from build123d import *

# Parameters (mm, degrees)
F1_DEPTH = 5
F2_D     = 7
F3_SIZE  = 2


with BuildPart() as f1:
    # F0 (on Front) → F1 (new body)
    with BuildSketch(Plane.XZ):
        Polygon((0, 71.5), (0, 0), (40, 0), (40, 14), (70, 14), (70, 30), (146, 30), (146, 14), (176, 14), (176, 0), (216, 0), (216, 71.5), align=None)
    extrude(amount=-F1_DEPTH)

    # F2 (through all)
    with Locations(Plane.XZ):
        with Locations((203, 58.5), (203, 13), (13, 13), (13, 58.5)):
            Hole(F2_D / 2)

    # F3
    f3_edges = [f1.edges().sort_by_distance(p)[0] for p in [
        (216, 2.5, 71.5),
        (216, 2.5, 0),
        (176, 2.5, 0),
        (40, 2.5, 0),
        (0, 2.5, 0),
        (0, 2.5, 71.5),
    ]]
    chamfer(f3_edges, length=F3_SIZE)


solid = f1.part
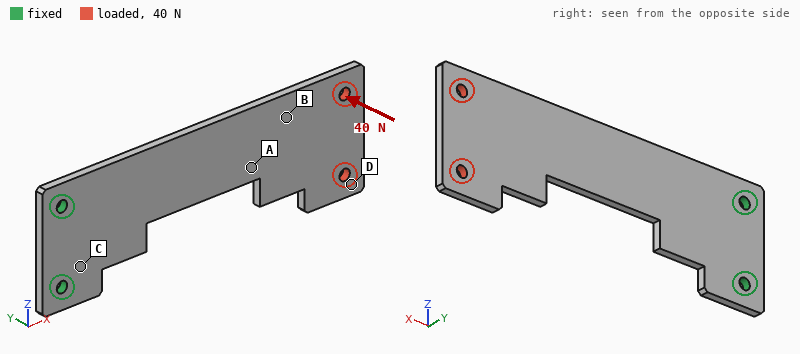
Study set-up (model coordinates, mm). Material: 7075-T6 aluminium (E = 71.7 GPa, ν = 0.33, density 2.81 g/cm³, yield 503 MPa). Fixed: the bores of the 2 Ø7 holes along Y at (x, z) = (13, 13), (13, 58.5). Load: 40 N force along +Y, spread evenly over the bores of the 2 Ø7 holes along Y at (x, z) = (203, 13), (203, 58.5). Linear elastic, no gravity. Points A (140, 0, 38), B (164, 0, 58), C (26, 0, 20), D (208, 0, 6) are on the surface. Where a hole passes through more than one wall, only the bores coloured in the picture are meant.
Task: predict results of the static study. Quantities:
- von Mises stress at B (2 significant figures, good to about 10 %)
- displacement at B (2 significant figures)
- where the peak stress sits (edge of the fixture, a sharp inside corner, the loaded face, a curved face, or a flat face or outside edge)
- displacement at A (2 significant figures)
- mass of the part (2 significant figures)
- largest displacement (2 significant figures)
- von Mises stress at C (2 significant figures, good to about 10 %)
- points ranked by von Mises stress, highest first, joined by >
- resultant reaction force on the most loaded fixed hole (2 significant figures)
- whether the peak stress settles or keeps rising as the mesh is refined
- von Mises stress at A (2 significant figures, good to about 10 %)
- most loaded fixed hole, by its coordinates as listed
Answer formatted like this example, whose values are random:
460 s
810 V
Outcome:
7.8 MPa
1.6 mm
edge of the fixture
1.2 mm
170 g
2.7 mm
21 MPa
C > A > B > D
24 N
keeps rising
16 MPa
(13, 58.5)
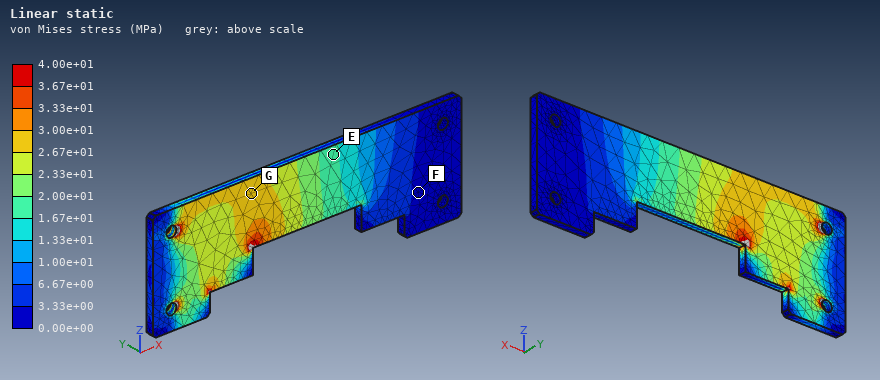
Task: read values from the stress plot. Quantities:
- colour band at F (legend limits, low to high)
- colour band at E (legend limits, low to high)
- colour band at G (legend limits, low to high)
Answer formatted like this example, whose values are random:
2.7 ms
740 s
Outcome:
0.00e+00 to 3.33e+00 MPa
1.67e+01 to 2.00e+01 MPa
2.67e+01 to 3.00e+01 MPa
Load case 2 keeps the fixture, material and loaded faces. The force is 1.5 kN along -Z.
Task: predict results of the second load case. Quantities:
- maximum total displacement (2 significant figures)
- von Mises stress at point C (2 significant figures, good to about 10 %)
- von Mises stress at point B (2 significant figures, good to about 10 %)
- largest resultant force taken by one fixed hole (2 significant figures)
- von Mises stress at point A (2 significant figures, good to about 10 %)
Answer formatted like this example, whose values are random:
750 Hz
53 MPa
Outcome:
1.2 mm
60 MPa
23 MPa
6.1 kN
37 MPa
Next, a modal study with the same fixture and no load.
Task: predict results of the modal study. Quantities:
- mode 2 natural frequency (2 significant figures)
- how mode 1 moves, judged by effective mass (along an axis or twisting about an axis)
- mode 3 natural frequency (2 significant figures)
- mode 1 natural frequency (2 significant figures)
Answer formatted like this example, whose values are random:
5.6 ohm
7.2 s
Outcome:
520 Hz
along Y
670 Hz
92 Hz
